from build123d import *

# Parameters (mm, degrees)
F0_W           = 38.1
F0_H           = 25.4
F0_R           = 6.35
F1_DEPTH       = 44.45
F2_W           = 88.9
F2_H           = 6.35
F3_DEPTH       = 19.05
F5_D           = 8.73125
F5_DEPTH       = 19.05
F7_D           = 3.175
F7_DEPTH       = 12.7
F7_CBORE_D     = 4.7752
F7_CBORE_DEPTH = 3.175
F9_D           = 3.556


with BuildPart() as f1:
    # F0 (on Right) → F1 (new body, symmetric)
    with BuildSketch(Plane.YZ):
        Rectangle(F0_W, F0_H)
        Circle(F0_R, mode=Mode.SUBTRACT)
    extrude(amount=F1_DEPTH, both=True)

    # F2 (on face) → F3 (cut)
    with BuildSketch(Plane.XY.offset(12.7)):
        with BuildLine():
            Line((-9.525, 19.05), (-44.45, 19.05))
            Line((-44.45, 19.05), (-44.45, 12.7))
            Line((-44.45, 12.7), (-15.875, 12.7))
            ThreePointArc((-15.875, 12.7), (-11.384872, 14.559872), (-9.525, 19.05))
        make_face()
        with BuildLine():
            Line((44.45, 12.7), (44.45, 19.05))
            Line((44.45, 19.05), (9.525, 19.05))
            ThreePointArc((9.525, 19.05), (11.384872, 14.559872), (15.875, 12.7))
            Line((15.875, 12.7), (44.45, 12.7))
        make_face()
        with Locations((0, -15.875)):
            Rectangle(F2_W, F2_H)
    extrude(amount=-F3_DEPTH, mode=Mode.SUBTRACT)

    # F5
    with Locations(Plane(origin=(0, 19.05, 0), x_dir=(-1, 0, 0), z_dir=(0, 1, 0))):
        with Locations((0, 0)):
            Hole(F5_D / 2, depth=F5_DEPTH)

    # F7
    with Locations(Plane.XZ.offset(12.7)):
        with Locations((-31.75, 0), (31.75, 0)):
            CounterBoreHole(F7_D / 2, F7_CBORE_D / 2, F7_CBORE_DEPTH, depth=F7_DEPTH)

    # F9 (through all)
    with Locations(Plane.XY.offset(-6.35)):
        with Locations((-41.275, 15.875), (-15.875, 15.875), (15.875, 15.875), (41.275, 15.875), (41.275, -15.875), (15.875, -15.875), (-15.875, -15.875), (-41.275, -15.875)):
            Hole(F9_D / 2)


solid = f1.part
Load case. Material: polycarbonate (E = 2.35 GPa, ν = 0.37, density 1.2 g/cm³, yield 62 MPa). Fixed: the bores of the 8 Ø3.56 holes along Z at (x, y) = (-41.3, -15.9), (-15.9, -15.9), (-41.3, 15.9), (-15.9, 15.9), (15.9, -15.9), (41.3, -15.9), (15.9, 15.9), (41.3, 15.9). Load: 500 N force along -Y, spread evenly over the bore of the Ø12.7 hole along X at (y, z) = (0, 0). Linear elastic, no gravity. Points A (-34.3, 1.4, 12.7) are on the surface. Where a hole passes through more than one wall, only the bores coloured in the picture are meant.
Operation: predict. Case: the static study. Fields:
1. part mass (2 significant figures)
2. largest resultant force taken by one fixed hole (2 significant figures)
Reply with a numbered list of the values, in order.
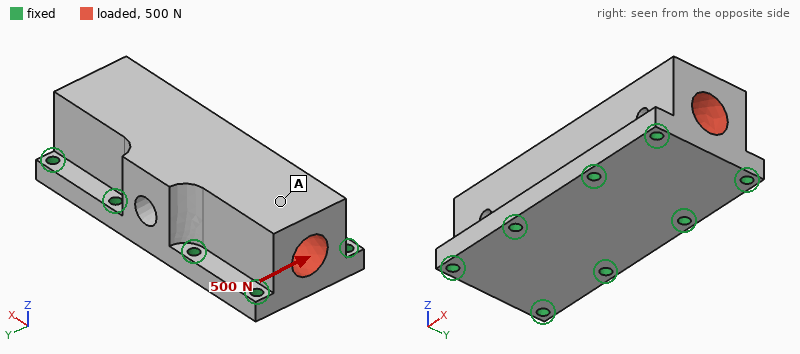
1. 65 g
2. 93 N
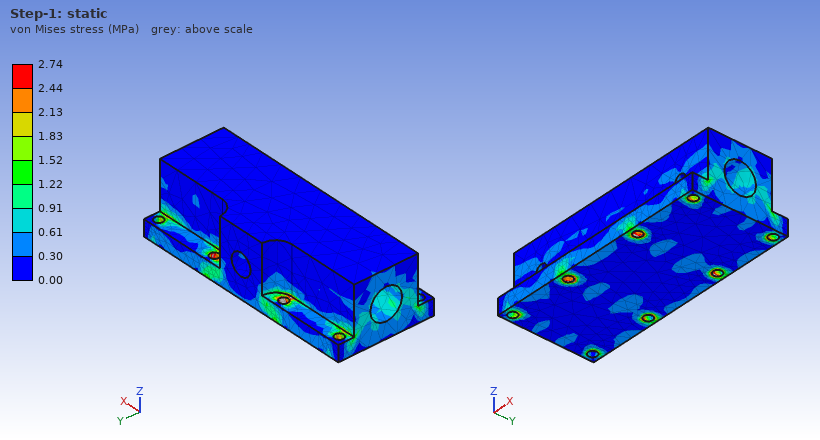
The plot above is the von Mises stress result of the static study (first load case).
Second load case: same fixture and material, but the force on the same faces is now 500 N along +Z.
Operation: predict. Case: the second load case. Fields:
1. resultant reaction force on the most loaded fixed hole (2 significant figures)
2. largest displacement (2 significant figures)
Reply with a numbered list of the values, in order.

1. 80 N
2. 12 µm
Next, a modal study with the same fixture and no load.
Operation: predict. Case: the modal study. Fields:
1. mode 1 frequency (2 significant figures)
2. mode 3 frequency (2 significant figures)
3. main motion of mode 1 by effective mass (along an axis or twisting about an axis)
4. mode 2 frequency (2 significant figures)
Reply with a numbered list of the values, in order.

1. 4000 Hz
2. 4900 Hz
3. along Y
4. 4700 Hz
